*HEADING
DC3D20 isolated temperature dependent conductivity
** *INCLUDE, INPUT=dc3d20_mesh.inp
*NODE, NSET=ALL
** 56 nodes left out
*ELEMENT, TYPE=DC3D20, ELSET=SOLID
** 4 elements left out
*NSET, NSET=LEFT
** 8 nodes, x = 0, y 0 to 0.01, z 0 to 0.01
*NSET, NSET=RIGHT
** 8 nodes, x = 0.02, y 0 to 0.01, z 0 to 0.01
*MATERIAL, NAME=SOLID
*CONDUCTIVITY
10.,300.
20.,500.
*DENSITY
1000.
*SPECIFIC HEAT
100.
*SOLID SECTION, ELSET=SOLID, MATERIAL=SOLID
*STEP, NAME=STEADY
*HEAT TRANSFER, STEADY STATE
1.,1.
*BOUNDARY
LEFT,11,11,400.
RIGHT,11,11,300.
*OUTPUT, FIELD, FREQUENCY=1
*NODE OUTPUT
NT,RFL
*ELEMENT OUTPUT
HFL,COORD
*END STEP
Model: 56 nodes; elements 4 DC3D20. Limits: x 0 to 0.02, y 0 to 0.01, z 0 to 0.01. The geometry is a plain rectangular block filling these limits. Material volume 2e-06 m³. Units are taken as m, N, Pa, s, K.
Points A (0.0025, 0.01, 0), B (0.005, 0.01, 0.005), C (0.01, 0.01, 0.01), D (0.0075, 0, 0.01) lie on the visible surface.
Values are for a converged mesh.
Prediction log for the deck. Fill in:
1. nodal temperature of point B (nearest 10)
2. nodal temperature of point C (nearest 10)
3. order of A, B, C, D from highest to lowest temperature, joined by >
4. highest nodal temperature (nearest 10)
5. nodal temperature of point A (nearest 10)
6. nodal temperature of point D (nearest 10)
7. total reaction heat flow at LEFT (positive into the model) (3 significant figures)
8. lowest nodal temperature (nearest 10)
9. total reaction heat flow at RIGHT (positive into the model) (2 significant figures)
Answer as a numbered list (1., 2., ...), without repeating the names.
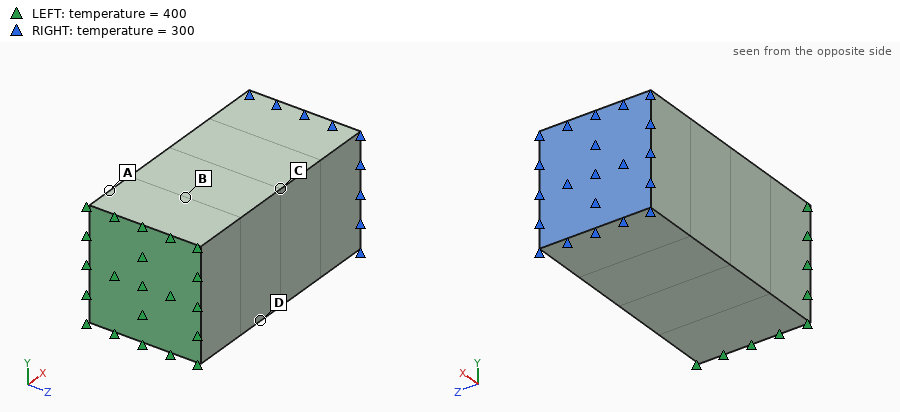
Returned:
1. 380 K
2. 350 K
3. A > B > D > C
4. 400 K
5. 390 K
6. 370 K
7. 6.25 W
8. 300 K
9. -6.3 W
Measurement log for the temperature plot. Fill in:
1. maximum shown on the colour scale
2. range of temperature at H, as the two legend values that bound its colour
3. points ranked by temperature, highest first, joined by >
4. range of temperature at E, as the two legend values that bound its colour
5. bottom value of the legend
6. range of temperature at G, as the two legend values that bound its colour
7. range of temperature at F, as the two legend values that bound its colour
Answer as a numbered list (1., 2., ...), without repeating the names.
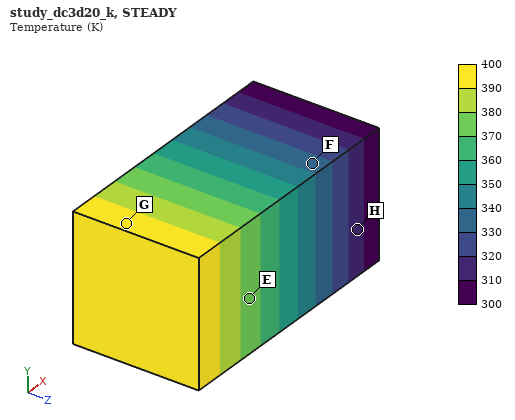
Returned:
1. 400 K
2. 310 to 320 K
3. G > E > F > H
4. 370 to 380 K
5. 300 K
6. 390 to 400 K
7. 330 to 340 K
